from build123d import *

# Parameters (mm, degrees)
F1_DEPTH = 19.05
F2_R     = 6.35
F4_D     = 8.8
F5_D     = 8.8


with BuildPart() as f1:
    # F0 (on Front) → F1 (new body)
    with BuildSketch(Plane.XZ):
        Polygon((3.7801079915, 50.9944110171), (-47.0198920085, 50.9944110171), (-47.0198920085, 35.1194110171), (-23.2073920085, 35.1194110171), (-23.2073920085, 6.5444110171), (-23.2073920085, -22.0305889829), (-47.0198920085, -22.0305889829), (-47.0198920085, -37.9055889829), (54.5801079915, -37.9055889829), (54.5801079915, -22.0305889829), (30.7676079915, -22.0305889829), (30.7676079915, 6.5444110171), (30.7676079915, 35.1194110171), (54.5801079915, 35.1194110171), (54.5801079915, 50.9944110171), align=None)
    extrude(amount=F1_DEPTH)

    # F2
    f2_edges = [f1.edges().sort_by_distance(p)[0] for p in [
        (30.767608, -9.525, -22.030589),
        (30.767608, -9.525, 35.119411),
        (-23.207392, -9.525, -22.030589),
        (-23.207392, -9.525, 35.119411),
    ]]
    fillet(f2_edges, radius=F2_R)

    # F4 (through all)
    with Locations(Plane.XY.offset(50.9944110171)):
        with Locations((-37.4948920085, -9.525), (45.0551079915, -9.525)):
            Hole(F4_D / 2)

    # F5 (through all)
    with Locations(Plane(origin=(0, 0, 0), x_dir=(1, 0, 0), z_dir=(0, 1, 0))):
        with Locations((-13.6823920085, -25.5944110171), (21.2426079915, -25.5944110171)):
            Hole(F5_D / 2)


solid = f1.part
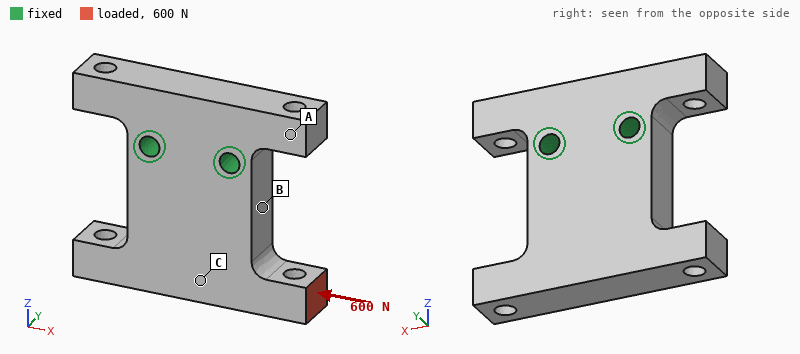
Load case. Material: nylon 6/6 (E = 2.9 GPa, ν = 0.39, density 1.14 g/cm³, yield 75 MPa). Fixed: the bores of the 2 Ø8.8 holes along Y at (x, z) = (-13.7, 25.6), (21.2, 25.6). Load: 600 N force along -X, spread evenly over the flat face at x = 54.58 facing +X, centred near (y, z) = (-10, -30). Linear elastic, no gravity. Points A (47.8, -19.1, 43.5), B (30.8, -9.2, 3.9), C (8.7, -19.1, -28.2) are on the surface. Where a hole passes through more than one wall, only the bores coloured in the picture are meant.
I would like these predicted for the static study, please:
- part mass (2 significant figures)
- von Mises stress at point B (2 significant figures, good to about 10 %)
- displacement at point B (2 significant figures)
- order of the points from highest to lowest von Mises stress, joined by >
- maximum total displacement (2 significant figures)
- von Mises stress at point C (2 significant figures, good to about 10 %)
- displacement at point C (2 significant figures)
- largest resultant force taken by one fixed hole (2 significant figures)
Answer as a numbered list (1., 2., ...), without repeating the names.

1. 130 g
2. 2.3 MPa
3. 0.034 mm
4. B > C > A
5. 0.17 mm
6. 1.4 MPa
7. 0.077 mm
8. 890 N
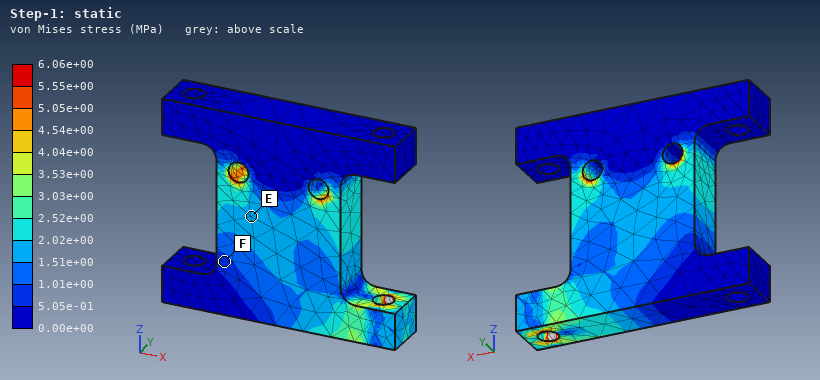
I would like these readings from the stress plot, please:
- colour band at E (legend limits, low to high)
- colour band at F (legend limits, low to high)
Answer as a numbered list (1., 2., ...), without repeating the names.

1. 1.51e+00 to 2.02e+00 MPa
2. 5.05e-01 to 1.01e+00 MPa
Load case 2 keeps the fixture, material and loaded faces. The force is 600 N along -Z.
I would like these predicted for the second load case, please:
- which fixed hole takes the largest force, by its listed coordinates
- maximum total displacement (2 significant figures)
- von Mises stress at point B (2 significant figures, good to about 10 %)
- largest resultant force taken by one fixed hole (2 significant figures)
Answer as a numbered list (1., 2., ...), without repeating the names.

1. (21.2, 25.6)
2. 0.57 mm
3. 3.9 MPa
4. 1.1 kN
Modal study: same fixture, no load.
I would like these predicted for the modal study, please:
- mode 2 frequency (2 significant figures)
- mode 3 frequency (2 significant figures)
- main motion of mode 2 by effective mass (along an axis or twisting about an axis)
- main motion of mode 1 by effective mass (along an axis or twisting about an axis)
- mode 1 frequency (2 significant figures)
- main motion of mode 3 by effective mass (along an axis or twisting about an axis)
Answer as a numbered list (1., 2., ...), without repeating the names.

1. 1400 Hz
2. 1900 Hz
3. twisting about Z
4. along Y
5. 940 Hz
6. along X
